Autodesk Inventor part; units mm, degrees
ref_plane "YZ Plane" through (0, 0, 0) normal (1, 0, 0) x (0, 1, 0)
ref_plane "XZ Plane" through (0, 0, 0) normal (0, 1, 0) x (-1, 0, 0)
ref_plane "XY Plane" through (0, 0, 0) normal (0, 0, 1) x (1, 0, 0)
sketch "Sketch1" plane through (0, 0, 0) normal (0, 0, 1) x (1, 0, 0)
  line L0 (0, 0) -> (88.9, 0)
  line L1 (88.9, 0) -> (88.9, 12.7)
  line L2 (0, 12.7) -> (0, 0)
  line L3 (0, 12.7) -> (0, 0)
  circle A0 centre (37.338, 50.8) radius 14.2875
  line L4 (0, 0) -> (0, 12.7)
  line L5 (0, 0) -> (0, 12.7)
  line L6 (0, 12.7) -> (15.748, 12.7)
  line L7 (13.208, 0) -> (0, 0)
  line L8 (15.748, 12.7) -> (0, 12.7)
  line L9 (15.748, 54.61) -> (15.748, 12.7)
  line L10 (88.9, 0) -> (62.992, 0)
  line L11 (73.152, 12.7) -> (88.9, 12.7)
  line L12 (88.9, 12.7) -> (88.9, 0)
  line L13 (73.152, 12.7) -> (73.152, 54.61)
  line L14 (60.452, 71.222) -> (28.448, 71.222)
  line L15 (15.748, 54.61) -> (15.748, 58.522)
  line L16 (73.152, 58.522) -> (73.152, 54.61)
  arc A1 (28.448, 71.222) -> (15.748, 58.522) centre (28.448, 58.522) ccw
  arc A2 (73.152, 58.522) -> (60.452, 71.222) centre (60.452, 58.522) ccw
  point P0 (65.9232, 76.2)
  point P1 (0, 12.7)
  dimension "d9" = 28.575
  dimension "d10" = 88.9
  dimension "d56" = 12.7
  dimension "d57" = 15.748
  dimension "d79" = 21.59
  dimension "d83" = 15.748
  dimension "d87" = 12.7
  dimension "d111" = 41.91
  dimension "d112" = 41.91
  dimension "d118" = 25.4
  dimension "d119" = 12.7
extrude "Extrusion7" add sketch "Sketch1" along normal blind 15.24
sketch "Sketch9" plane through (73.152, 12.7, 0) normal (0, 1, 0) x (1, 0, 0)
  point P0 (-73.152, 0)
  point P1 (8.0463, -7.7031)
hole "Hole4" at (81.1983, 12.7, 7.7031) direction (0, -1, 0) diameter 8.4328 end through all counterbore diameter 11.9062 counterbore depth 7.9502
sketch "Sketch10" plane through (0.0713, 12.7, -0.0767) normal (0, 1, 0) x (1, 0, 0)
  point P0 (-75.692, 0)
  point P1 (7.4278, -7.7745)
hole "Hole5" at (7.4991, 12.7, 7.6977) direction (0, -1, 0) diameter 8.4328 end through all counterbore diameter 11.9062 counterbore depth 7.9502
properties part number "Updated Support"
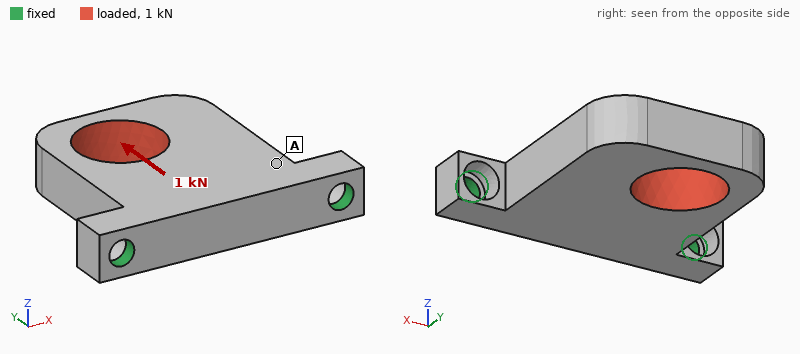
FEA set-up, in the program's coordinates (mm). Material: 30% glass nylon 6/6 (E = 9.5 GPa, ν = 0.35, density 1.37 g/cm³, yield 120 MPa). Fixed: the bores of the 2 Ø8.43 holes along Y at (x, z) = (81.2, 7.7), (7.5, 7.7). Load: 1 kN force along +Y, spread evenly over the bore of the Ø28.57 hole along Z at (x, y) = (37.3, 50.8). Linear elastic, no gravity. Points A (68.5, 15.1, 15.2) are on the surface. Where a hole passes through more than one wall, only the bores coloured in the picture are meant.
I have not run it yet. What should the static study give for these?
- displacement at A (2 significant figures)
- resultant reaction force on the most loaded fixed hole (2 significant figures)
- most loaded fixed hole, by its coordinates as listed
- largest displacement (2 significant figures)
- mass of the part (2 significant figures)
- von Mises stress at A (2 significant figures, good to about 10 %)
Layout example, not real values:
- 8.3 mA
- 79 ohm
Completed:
- 14 µm
- 680 N
- (7.5, 7.7)
- 44 µm
- 76 g
- 2.9 MPa
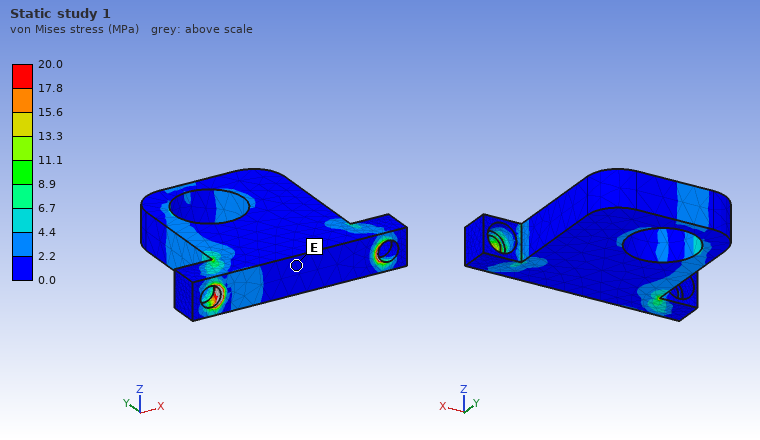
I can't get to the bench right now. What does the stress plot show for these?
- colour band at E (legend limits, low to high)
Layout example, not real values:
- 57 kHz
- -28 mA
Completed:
- 0.0 to 2.2 MPa
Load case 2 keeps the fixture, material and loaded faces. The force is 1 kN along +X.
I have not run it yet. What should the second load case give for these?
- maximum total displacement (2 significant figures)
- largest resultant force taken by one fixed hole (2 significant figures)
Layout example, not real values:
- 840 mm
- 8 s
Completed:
- 0.11 mm
- 890 N
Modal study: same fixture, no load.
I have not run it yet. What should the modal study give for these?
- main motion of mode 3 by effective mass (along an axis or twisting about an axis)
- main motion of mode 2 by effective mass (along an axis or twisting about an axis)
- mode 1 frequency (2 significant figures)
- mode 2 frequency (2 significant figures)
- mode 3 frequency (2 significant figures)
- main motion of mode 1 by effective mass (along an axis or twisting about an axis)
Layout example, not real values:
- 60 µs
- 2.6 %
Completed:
- along X
- twisting about Y
- 660 Hz
- 2800 Hz
- 2900 Hz
- along Z
